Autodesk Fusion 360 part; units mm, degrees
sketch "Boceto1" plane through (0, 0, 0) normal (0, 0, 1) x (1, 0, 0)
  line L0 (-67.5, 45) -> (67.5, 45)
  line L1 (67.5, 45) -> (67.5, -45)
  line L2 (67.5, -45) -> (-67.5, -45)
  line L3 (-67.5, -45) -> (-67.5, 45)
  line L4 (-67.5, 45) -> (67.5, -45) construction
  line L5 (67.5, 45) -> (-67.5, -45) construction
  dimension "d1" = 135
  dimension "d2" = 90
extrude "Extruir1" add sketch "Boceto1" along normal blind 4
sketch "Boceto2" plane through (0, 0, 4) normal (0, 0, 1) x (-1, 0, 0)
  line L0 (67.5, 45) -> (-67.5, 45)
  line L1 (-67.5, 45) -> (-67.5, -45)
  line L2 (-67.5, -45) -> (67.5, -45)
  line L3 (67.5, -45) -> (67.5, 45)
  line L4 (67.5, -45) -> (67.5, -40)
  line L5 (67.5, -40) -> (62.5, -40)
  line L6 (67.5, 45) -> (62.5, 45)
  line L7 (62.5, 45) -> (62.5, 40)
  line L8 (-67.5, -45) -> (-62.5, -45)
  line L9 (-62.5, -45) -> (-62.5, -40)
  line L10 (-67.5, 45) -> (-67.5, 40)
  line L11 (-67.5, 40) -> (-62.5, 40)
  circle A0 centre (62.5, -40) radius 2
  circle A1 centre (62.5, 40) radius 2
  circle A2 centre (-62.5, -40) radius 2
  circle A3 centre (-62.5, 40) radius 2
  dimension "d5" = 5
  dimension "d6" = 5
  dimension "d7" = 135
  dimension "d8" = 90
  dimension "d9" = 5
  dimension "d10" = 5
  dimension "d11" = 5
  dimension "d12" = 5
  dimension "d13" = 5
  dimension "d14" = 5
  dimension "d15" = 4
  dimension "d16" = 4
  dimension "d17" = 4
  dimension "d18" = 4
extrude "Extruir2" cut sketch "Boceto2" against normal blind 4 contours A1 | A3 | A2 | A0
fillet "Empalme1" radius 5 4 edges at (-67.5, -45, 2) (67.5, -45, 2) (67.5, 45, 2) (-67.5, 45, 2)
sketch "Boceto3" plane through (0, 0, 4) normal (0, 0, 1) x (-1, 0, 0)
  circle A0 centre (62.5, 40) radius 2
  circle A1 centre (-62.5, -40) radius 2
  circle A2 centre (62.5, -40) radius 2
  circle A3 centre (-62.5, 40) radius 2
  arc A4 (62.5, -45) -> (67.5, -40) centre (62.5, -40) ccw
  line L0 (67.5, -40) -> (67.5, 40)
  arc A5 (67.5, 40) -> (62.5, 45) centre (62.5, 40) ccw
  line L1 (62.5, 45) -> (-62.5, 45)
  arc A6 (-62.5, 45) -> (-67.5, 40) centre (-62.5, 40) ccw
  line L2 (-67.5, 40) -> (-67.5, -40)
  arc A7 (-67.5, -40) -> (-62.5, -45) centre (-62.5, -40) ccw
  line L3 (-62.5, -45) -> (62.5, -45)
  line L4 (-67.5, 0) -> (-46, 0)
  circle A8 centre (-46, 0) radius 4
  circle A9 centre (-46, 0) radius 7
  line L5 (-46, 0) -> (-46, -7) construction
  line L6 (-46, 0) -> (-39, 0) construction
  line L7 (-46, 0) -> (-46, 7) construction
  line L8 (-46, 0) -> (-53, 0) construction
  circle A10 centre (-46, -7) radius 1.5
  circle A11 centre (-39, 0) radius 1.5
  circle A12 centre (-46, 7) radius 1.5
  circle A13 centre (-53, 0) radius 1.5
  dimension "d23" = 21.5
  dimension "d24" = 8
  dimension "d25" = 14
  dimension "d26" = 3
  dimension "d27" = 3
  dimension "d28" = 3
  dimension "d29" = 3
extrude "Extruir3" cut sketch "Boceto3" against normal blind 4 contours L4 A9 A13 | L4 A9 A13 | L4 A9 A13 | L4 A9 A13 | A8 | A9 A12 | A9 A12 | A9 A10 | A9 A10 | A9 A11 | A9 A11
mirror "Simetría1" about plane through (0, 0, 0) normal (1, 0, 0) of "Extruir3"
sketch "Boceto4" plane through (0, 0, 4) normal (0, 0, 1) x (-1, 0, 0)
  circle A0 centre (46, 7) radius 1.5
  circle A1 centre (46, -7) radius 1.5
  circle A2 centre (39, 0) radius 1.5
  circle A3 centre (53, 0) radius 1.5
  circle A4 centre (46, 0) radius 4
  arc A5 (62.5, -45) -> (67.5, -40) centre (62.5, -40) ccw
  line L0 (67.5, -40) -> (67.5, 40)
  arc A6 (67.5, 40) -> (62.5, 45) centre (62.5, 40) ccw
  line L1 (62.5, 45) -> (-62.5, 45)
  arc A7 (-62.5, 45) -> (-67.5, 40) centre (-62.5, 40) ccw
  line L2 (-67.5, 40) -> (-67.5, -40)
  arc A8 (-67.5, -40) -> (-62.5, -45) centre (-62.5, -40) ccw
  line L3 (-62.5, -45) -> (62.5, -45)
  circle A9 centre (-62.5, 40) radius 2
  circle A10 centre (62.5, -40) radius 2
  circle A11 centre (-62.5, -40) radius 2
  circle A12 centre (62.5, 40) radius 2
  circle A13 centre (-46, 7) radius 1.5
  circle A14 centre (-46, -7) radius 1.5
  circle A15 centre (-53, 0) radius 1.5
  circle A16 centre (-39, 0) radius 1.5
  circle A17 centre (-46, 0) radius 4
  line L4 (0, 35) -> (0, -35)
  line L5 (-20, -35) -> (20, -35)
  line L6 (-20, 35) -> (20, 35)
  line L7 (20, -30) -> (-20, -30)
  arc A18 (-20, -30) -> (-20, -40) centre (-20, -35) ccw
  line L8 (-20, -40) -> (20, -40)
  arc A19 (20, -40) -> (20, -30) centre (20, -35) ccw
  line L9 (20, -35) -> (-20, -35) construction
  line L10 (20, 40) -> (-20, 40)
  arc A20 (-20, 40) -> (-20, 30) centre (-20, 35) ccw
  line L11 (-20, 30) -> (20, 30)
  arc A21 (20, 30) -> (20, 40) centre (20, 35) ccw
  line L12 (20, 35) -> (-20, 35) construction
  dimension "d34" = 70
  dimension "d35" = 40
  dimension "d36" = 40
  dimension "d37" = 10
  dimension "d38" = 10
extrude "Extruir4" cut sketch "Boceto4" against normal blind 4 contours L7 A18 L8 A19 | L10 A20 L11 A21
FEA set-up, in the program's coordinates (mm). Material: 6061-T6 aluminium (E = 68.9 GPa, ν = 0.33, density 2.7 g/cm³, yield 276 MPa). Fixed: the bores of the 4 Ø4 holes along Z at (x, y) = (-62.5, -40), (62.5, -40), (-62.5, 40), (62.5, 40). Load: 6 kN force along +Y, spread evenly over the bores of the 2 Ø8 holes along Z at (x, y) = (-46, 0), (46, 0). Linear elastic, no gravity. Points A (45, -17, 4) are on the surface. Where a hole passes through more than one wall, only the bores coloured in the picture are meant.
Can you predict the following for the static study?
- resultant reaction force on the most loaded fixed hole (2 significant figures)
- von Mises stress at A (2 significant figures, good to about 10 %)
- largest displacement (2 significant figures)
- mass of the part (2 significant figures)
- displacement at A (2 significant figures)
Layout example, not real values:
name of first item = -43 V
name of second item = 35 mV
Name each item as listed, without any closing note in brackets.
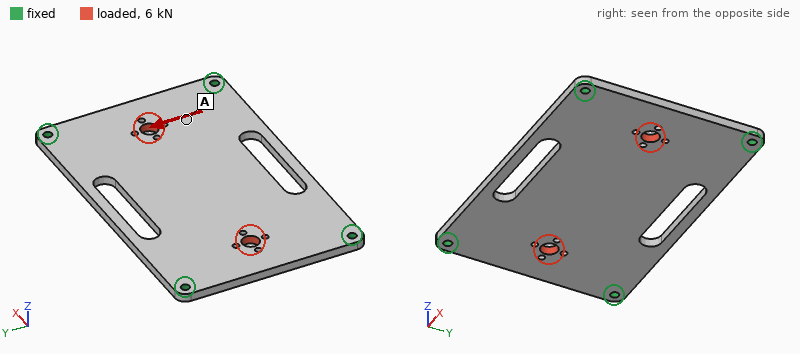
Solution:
resultant reaction force on the most loaded fixed hole = 1.6 kN
von Mises stress at A = 15 MPa
largest displacement = 17 µm
mass of the part = 120 g
displacement at A = 11 µm
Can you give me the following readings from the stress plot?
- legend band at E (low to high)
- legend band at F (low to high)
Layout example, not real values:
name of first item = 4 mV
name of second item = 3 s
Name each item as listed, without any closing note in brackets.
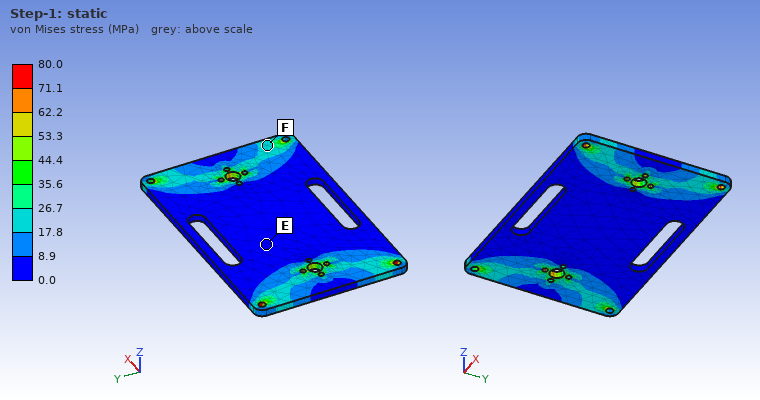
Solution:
legend band at E = 0.0 to 8.9 MPa
legend band at F = 17.8 to 26.7 MPa
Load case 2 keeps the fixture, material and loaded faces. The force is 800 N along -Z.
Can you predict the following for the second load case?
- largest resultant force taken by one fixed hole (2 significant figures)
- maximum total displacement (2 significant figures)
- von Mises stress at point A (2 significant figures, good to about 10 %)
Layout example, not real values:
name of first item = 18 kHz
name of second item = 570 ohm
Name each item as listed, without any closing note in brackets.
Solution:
largest resultant force taken by one fixed hole = 200 N
maximum total displacement = 0.17 mm
von Mises stress at point A = 13 MPa
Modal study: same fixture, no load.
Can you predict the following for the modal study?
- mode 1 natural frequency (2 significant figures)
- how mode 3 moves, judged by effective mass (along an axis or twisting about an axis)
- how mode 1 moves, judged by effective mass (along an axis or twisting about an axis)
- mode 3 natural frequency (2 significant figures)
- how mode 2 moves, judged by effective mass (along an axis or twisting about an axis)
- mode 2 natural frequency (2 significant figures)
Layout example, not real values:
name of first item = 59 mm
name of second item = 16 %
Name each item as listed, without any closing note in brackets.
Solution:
mode 1 natural frequency = 1000 Hz
how mode 3 moves, judged by effective mass = twisting about Y
how mode 1 moves, judged by effective mass = along Z
mode 3 natural frequency = 2500 Hz
how mode 2 moves, judged by effective mass = twisting about X
mode 2 natural frequency = 1900 Hz
